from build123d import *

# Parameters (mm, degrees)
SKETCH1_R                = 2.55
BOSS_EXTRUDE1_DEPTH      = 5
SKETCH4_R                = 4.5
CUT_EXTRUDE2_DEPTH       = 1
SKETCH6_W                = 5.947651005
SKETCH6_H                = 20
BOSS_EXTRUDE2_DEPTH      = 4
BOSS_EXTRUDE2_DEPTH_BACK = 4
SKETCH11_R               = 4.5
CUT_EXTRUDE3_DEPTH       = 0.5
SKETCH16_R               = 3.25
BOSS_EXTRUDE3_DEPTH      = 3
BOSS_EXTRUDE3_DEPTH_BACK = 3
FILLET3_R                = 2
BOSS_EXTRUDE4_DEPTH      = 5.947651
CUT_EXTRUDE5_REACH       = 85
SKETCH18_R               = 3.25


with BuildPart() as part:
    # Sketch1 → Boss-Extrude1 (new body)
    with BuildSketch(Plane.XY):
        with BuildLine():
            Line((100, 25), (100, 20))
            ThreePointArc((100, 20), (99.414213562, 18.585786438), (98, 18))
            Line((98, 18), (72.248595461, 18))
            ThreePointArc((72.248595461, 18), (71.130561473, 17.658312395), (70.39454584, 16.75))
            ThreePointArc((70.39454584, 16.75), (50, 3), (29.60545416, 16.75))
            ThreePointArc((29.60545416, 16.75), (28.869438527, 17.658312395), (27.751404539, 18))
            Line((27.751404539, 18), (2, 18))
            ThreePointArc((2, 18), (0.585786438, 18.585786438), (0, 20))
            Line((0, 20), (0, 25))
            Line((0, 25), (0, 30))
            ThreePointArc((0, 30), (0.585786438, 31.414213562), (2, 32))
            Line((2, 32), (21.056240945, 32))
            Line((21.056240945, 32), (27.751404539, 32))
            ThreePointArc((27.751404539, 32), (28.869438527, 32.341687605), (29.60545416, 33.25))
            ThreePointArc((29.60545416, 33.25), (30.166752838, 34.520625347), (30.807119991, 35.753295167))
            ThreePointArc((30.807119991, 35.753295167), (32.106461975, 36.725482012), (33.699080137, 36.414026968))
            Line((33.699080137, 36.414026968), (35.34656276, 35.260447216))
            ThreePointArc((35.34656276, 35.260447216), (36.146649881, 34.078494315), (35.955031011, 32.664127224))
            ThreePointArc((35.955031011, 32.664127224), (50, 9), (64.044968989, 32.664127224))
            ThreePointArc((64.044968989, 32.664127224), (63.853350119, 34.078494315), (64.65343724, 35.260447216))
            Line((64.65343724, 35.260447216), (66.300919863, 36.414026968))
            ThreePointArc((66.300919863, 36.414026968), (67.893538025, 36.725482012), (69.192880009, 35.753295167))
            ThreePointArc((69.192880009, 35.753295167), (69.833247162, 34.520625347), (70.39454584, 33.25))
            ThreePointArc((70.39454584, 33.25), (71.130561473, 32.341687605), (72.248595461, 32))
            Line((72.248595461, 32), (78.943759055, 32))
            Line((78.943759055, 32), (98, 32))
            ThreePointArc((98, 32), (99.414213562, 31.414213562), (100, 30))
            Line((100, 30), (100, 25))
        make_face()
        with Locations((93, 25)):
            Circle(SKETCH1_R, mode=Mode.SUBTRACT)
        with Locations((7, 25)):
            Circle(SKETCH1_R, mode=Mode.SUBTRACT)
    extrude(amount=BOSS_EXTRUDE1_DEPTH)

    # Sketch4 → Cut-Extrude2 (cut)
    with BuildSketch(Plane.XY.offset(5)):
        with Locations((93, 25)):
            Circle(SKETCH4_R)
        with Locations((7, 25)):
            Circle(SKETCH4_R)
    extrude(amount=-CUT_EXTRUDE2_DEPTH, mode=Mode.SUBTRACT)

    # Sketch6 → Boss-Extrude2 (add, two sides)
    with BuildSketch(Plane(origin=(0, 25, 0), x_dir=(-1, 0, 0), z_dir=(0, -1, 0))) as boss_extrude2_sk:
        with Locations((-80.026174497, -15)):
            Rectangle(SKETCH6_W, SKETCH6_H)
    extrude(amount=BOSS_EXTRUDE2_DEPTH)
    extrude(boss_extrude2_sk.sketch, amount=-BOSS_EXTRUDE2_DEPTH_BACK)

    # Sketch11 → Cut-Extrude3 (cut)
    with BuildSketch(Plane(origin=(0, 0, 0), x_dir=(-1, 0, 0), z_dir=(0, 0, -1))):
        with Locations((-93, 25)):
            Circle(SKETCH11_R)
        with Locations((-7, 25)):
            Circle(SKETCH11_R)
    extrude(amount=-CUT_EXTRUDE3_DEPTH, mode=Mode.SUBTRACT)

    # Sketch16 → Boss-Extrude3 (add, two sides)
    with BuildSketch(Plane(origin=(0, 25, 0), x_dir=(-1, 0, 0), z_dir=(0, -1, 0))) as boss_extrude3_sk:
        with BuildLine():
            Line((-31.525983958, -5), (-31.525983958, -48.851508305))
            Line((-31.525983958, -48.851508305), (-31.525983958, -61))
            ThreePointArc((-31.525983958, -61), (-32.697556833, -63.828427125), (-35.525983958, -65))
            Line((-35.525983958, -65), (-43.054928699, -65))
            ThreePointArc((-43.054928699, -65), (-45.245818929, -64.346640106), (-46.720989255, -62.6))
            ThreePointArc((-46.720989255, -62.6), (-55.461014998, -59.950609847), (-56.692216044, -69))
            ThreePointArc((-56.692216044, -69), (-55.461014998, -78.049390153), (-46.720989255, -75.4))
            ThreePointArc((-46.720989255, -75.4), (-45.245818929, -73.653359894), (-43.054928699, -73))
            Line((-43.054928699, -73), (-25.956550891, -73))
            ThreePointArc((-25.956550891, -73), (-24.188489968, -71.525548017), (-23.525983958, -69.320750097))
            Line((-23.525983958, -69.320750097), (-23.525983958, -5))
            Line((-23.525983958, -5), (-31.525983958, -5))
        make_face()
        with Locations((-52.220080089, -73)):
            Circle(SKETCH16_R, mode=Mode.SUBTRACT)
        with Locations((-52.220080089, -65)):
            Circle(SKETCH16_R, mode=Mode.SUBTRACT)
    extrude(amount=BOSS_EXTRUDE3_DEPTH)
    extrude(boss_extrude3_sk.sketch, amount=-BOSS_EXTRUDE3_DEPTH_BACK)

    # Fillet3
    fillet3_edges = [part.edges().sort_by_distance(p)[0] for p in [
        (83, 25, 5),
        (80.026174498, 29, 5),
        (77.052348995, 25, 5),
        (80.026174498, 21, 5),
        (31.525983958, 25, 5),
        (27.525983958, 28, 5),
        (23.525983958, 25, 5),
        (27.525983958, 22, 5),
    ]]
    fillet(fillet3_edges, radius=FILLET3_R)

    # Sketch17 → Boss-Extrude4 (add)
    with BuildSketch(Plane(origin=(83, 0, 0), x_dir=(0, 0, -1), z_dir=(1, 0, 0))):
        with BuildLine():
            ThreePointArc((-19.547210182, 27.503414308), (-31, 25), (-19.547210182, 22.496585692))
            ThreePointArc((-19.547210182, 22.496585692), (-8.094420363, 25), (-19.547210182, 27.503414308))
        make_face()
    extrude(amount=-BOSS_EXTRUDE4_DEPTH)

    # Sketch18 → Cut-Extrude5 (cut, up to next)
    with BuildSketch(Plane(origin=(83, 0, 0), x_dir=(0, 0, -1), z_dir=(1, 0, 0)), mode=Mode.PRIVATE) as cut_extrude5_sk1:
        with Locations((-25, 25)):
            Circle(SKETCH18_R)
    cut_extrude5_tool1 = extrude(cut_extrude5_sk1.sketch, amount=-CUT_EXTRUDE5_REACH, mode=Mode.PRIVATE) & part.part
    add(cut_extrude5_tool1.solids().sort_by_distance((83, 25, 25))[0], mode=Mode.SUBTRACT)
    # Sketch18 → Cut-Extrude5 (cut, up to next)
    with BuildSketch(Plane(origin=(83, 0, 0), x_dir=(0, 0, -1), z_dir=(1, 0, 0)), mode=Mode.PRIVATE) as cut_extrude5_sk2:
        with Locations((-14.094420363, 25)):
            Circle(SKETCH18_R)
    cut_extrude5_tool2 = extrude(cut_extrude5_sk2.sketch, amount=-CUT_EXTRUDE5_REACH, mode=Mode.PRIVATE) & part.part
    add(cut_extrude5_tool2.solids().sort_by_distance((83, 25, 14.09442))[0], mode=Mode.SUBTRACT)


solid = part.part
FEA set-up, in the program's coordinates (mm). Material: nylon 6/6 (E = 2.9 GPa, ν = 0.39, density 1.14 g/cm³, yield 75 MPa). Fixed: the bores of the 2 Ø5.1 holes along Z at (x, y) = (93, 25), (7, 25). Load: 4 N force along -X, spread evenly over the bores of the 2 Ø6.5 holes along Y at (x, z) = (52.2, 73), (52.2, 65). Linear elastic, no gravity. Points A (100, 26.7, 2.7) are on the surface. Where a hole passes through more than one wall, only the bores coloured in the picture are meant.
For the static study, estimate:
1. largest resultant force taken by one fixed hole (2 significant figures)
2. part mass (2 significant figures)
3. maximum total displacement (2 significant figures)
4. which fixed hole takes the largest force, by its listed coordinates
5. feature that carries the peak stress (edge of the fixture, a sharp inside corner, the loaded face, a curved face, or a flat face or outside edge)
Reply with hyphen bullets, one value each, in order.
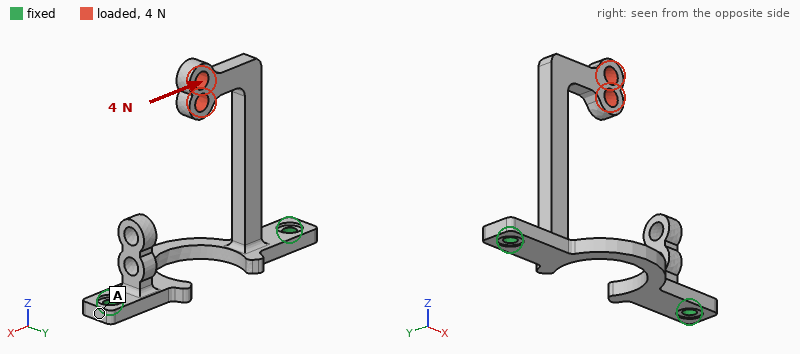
- 4.6 N
- 14 g
- 1.3 mm
- (7, 25)
- a curved face
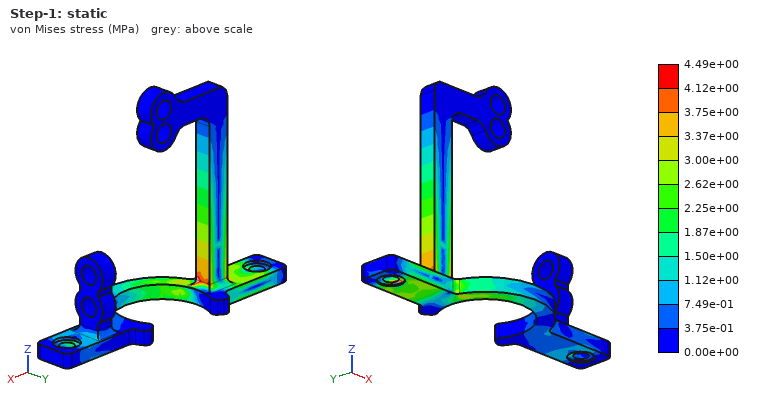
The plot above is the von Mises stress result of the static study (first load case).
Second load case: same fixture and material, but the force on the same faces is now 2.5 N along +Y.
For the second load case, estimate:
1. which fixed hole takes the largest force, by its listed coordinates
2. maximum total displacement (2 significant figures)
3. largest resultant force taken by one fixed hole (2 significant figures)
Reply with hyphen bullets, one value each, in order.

- (7, 25)
- 1.4 mm
- 2.3 N
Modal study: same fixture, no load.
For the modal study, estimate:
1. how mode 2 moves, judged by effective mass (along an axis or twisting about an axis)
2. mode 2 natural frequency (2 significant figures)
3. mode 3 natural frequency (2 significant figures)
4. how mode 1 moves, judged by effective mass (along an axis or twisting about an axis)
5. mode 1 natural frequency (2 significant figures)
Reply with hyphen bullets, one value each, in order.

- along X
- 170 Hz
- 590 Hz
- along Y
- 150 Hz
